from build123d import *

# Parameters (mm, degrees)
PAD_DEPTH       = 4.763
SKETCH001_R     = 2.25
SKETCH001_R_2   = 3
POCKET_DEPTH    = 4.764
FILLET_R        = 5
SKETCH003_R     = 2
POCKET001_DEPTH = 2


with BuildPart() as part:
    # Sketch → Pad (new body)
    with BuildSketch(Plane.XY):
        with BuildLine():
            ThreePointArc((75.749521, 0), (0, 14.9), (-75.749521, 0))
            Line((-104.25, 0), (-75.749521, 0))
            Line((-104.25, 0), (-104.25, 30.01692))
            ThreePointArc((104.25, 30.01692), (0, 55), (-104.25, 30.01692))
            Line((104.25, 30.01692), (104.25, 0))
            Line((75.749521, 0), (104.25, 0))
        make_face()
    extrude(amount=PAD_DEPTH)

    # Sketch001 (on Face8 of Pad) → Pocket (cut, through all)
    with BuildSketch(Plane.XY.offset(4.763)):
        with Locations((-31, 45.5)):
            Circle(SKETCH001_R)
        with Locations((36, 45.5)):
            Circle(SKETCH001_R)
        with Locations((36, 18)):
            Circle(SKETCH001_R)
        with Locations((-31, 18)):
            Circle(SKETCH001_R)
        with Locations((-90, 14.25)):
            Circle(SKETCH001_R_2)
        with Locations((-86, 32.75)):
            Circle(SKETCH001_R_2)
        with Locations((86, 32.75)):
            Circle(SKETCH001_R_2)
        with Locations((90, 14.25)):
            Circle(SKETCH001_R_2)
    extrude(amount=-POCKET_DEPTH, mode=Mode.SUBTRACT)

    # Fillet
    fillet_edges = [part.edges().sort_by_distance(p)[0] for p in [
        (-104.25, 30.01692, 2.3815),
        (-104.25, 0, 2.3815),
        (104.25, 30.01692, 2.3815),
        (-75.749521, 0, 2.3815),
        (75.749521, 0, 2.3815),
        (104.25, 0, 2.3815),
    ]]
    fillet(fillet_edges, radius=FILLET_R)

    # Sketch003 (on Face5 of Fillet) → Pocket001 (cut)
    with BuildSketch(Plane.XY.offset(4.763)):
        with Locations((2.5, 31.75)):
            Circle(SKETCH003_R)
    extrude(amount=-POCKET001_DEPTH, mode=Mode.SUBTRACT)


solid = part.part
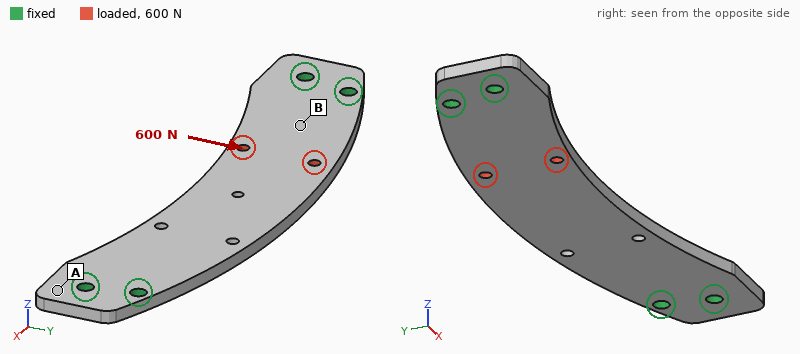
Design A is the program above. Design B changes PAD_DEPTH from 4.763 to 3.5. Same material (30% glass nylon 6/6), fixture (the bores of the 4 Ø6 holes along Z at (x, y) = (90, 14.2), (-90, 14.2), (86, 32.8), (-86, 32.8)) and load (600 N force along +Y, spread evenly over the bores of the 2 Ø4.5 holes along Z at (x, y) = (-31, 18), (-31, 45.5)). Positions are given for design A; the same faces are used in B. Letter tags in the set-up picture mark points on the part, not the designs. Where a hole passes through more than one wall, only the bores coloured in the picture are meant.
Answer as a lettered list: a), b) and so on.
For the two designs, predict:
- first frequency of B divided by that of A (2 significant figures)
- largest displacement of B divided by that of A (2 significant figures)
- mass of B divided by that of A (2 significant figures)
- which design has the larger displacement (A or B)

a) 0.74
b) 1.4
c) 0.74
d) B
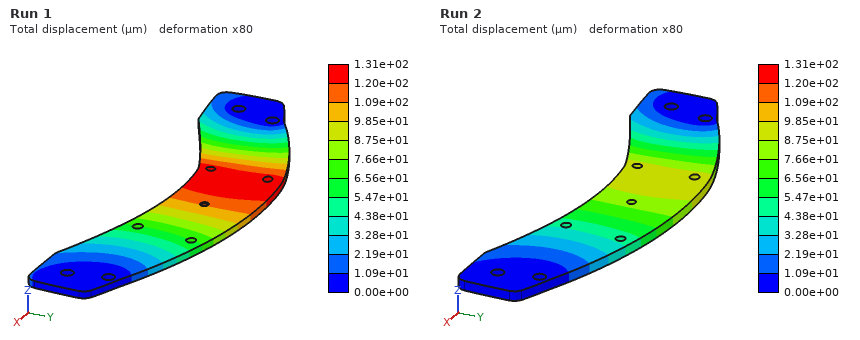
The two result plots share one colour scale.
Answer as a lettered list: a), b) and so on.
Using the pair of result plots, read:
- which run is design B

a) Run 1
